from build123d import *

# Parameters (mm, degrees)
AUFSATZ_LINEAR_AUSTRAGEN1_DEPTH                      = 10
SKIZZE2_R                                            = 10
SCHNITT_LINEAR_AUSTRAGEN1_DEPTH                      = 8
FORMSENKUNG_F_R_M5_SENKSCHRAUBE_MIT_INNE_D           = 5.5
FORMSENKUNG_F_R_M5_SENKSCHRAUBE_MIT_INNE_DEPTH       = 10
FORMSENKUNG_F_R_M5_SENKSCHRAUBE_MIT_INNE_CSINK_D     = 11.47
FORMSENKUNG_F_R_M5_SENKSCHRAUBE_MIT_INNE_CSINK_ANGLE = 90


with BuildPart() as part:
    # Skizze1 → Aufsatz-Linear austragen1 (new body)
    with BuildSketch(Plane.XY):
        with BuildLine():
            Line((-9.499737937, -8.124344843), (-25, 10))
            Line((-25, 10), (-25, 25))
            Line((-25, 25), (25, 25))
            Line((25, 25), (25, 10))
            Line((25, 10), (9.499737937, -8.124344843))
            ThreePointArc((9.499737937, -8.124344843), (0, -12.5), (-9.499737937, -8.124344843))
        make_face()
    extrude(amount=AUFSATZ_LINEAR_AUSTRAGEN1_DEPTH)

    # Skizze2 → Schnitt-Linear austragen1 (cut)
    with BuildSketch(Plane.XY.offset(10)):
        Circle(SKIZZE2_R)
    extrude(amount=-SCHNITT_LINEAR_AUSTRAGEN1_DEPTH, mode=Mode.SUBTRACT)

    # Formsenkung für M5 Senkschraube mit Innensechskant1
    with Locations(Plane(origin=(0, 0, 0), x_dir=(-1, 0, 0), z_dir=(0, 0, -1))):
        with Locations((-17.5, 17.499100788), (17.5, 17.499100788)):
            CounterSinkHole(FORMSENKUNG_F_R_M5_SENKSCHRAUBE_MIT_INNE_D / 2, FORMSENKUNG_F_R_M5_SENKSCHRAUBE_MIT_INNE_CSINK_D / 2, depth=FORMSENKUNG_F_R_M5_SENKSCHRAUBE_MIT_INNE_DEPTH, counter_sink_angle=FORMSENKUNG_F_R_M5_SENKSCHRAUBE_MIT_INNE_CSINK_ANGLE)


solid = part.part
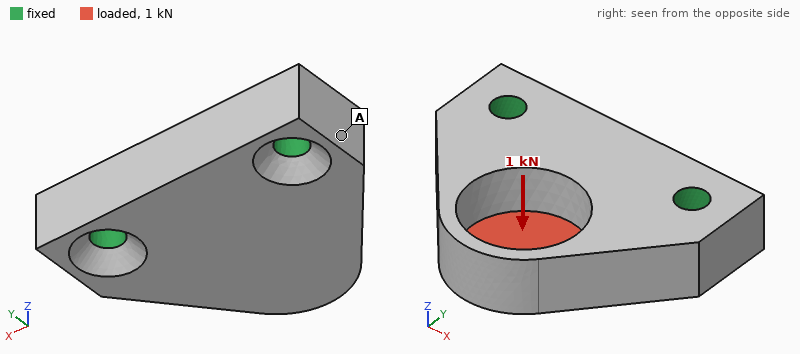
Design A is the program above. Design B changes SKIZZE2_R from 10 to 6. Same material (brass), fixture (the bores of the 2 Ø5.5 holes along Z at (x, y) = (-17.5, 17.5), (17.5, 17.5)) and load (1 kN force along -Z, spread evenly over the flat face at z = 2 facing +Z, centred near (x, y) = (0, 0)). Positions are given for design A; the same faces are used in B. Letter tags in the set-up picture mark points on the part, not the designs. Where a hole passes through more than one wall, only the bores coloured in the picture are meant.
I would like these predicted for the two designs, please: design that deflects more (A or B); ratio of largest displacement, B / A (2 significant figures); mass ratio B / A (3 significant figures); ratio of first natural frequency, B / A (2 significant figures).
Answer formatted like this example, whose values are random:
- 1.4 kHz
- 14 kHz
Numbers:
- A
- 0.80
- 1.14
- 0.88
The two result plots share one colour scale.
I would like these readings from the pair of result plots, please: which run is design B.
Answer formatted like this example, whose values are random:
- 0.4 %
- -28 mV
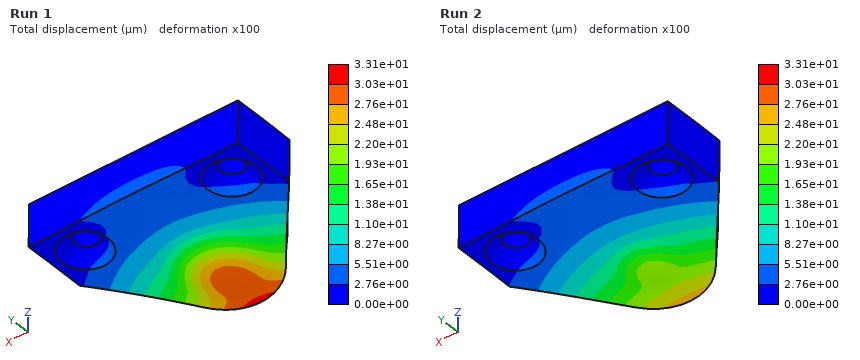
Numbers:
- Run 2
